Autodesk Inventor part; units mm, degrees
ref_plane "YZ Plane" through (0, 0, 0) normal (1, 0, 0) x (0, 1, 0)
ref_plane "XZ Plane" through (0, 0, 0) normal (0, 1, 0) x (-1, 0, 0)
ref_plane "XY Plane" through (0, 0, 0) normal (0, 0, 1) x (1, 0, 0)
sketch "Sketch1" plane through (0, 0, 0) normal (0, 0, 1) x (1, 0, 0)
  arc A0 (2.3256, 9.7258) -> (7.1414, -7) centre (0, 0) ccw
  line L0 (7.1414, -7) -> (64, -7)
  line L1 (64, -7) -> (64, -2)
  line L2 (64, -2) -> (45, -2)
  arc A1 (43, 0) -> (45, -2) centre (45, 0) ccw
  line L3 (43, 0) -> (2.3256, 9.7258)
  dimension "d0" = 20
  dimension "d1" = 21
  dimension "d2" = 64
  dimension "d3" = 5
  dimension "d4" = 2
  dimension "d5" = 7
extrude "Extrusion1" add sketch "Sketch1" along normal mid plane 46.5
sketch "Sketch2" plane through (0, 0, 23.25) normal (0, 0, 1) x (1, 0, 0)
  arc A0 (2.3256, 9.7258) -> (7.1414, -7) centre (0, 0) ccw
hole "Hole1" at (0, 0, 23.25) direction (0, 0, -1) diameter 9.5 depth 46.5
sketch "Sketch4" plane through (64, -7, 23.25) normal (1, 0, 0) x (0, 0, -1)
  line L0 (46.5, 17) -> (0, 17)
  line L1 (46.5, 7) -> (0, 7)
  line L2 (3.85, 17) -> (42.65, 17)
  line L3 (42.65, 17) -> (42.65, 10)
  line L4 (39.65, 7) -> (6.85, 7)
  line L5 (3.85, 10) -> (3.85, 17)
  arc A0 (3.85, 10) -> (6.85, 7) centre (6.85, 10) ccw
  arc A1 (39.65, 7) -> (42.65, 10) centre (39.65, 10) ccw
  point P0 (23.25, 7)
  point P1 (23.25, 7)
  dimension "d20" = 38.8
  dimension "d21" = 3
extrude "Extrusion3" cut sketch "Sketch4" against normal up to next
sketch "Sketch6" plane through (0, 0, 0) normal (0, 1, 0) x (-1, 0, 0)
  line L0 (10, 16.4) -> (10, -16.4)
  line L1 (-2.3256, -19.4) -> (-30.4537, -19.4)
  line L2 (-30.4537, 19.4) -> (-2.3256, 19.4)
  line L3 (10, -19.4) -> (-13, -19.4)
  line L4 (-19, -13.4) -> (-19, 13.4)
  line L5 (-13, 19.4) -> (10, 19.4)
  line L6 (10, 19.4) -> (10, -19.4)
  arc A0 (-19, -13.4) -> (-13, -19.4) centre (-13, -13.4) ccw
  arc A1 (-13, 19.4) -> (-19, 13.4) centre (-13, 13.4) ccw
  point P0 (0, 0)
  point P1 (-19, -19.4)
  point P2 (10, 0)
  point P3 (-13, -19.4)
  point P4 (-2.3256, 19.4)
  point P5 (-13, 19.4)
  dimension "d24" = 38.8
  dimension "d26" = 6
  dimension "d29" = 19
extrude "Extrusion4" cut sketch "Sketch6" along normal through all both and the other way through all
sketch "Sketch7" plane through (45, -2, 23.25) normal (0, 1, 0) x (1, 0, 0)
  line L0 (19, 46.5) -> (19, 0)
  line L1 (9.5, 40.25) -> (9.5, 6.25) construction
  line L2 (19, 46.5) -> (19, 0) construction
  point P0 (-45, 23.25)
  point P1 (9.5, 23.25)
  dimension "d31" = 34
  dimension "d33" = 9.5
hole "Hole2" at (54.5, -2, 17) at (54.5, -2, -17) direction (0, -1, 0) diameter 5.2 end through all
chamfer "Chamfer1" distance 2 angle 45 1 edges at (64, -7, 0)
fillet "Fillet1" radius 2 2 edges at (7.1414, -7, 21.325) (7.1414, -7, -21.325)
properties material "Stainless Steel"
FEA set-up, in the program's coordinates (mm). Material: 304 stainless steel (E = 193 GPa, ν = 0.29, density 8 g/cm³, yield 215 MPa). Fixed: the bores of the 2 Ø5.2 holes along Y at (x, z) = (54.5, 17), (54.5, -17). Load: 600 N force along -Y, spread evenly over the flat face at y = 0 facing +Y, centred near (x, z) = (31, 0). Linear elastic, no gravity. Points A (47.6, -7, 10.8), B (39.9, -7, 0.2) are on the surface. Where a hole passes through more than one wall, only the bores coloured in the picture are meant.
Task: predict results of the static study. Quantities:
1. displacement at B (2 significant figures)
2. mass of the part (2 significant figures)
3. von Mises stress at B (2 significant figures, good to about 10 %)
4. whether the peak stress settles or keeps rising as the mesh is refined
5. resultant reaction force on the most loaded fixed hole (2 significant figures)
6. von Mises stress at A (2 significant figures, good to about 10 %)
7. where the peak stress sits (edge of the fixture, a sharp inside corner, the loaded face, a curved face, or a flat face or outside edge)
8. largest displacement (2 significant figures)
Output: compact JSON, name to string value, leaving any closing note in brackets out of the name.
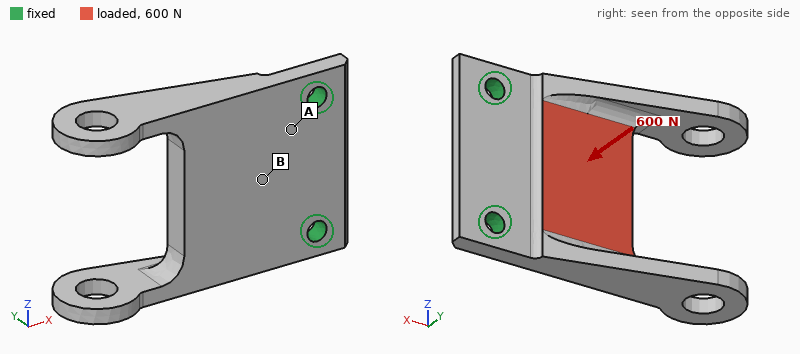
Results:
{"displacement at B": "16 µm", "mass of the part": "130 g", "von Mises stress at B": "19 MPa", "whether the peak stress settles or keeps rising as the mesh is refined": "keeps rising", "resultant reaction force on the most loaded fixed hole": "300 N", "von Mises stress at A": "45 MPa", "where the peak stress sits": "edge of the fixture", "largest displacement": "93 µm"}
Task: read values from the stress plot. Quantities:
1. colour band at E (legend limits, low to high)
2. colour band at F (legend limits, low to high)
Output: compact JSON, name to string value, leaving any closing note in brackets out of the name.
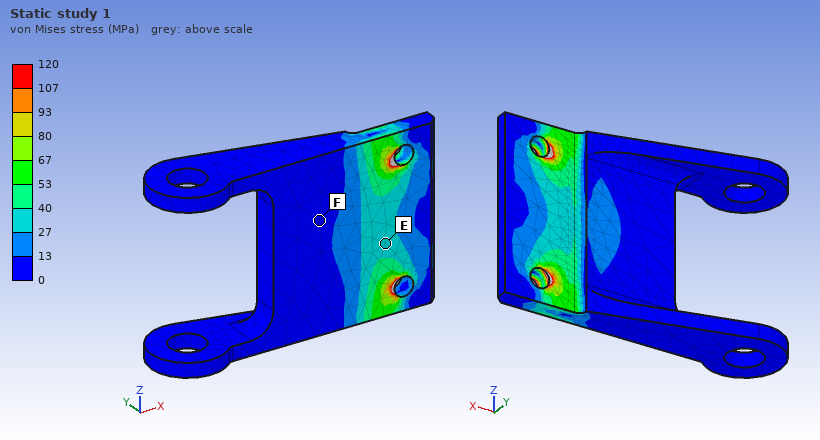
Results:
{"colour band at E": "27 to 40 MPa", "colour band at F": "0 to 13 MPa"}
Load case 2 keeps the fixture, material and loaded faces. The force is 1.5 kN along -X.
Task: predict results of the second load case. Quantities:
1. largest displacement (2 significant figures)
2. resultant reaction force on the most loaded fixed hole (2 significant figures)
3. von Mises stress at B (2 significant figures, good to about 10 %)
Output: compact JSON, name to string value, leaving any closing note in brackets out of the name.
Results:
{"largest displacement": "59 µm", "resultant reaction force on the most loaded fixed hole": "760 N", "von Mises stress at B": "10 MPa"}
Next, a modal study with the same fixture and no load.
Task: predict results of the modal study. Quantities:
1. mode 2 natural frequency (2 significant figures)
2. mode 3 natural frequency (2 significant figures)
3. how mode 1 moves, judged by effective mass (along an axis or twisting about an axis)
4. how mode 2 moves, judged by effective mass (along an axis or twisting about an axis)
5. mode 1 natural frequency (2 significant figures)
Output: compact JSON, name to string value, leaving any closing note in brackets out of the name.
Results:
{"mode 2 natural frequency": "2900 Hz", "mode 3 natural frequency": "3600 Hz", "how mode 1 moves, judged by effective mass": "along Y", "how mode 2 moves, judged by effective mass": "twisting about X", "mode 1 natural frequency": "1500 Hz"}
